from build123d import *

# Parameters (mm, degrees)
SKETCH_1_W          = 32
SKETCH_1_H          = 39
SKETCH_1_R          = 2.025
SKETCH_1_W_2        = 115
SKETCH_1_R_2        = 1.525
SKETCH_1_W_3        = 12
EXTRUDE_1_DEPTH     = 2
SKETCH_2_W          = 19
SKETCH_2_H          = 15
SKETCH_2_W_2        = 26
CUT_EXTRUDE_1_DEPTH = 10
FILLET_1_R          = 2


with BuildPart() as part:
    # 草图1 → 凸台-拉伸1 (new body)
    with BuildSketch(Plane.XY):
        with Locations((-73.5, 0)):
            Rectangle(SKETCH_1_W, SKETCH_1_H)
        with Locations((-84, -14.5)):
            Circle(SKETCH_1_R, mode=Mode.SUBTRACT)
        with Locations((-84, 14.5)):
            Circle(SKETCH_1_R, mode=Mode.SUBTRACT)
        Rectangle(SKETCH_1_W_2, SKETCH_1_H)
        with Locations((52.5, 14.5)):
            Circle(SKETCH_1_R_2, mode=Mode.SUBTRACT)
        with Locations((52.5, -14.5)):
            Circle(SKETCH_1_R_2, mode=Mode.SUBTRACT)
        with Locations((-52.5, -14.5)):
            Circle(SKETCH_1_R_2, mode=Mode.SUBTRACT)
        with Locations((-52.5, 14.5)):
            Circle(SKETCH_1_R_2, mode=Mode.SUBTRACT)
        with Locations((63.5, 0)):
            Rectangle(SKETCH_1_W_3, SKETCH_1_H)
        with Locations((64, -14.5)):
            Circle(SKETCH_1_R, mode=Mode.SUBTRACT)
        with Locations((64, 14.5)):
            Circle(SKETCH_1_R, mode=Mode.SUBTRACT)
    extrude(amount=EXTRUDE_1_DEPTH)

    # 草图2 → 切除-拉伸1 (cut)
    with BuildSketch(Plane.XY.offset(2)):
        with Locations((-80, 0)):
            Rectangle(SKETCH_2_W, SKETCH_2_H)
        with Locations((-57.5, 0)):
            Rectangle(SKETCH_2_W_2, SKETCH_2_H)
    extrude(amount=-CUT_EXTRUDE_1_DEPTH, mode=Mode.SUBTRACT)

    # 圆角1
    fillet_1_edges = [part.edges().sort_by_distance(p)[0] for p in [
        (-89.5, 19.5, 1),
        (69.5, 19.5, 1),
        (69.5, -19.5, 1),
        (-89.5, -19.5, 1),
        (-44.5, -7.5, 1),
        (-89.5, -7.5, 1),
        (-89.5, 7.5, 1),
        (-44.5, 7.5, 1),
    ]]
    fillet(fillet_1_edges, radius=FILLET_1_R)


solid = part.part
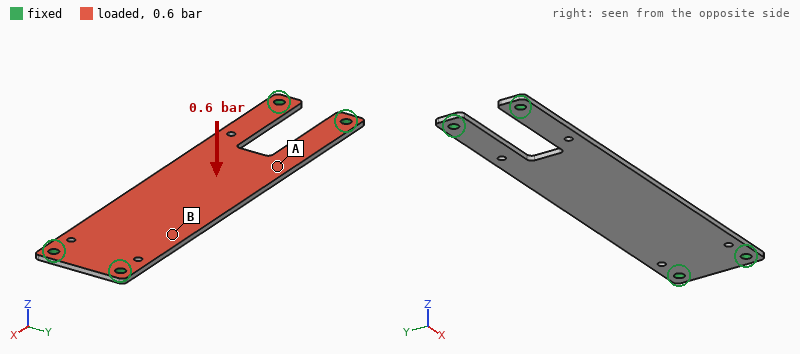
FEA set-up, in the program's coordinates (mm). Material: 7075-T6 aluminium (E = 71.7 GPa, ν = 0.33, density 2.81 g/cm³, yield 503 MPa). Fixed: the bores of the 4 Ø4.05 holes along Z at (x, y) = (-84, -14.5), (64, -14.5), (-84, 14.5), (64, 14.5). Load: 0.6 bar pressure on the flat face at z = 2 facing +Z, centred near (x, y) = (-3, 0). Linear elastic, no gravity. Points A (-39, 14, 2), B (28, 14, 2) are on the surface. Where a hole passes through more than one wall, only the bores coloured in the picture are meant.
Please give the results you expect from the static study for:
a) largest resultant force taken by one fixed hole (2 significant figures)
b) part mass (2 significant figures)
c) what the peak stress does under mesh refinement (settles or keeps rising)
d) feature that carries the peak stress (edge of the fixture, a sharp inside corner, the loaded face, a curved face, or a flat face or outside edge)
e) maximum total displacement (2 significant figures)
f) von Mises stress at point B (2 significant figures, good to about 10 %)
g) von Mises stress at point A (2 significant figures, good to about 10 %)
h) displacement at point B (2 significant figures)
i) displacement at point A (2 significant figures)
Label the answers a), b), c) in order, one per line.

a) 93 N
b) 31 g
c) keeps rising
d) edge of the fixture
e) 1.7 mm
f) 23 MPa
g) 57 MPa
h) 0.87 mm
i) 1.2 mm
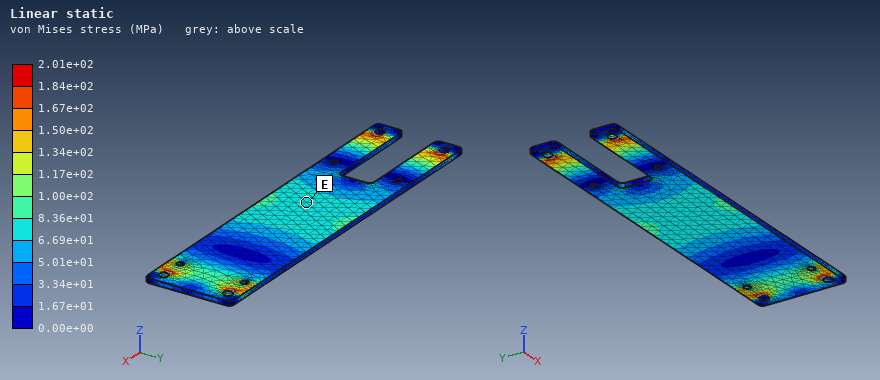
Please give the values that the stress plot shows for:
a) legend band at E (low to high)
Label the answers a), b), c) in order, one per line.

a) 6.69e+01 to 8.36e+01 MPa
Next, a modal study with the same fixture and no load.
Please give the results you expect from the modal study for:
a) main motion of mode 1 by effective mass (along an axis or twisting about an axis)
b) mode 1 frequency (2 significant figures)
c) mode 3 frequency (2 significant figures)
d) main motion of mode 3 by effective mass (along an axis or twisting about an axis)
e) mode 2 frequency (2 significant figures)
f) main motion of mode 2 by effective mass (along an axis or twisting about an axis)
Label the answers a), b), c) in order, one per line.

a) along Z
b) 460 Hz
c) 1300 Hz
d) twisting about Y
e) 1100 Hz
f) twisting about X
